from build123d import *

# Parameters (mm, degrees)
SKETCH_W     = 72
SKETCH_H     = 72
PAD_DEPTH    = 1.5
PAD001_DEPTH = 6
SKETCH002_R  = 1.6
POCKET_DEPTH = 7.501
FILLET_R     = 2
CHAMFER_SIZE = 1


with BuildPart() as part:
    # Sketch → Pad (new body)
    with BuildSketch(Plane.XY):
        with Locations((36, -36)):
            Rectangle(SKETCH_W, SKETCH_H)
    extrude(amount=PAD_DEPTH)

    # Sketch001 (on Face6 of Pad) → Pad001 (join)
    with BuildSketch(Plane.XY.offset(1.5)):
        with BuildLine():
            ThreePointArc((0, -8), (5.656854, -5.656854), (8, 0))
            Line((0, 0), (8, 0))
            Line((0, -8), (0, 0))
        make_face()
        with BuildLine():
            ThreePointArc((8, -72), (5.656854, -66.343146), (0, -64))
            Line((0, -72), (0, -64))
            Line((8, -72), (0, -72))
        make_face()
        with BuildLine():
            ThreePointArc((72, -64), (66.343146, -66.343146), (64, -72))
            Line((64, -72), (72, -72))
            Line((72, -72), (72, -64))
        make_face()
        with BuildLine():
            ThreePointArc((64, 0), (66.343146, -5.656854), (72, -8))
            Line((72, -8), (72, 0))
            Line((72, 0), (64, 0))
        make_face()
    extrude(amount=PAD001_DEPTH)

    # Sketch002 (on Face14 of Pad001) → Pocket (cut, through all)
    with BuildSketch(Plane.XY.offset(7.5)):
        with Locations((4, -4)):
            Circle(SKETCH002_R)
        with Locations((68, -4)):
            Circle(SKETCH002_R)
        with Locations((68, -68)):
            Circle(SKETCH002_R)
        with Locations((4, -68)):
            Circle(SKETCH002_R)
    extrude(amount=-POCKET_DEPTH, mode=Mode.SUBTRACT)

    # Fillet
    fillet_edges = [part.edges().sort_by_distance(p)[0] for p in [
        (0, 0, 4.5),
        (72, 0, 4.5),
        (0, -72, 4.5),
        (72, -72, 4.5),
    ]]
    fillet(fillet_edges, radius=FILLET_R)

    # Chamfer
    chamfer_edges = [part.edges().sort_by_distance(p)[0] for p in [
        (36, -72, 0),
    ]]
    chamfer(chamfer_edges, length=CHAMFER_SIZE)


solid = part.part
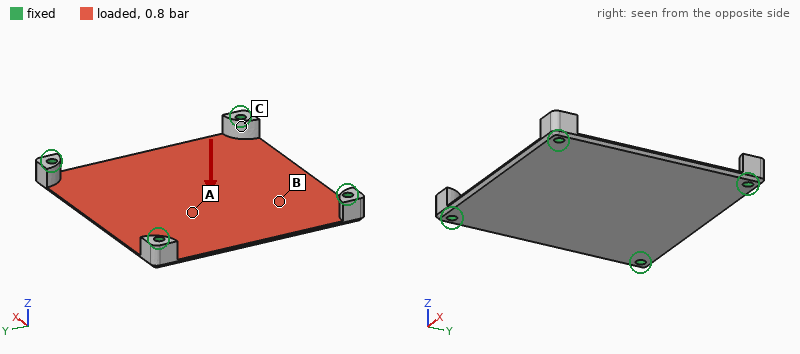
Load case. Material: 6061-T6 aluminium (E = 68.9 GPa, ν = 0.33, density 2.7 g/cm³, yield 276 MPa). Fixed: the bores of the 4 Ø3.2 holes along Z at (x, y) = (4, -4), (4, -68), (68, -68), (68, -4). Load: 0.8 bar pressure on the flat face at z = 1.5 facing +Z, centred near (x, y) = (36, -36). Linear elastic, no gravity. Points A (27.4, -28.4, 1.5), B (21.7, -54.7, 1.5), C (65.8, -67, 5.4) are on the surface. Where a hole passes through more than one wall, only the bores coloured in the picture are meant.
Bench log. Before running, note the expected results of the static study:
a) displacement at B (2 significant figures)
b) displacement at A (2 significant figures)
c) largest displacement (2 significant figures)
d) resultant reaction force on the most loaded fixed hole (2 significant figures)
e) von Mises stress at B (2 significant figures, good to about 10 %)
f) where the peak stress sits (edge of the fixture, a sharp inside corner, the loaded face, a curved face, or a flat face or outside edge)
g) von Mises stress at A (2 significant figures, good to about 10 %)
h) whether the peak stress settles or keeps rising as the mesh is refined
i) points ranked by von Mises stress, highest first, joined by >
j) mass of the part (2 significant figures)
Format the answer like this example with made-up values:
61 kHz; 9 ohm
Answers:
0.28 mm; 0.41 mm; 0.45 mm; 110 N; 27 MPa; edge of the fixture; 42 MPa; keeps rising; A > B > C; 23 g
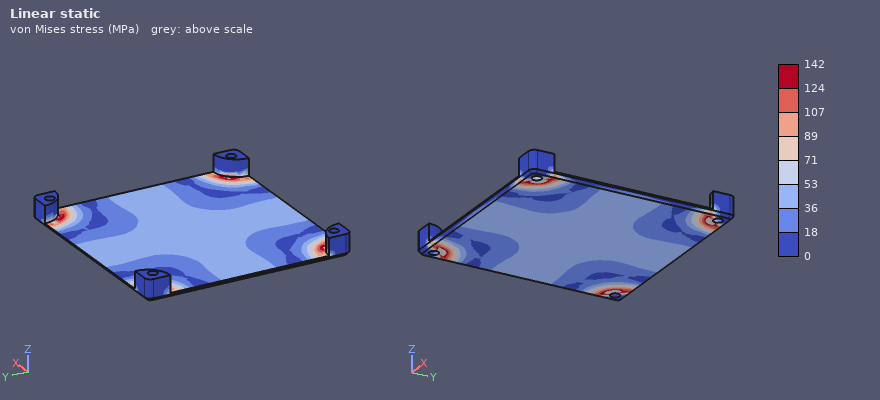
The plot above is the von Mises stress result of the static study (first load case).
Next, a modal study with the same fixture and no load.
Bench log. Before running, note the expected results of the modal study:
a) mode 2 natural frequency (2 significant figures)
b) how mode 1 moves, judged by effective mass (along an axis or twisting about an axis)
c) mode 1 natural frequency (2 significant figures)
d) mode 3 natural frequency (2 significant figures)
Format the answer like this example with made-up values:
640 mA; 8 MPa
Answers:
2300 Hz; along Z; 1300 Hz; 2300 Hz
